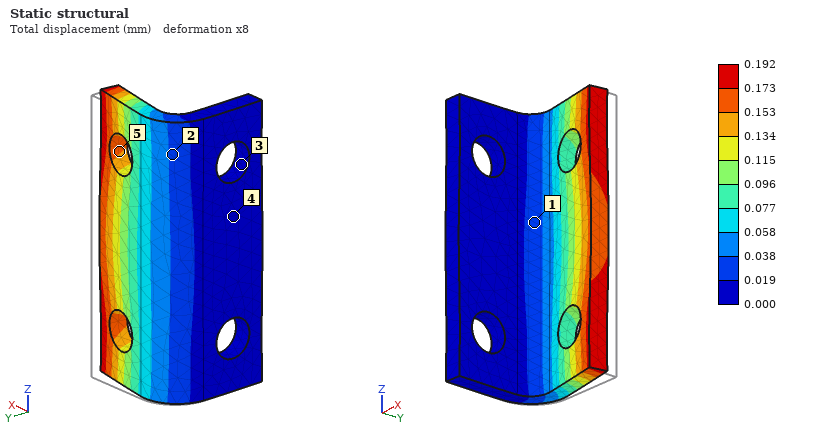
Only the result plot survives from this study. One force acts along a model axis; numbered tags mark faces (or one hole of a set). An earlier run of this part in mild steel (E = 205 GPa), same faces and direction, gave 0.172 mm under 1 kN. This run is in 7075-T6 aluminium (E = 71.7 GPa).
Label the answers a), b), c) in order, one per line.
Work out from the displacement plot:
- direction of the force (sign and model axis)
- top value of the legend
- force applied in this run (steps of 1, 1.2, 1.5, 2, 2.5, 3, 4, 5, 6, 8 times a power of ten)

a) -Y
b) 0.192 mm
c) 400 N
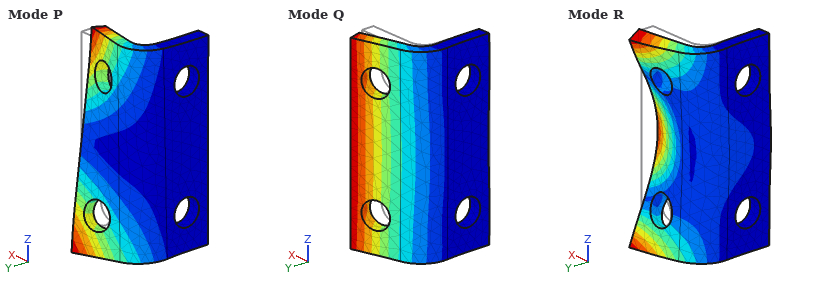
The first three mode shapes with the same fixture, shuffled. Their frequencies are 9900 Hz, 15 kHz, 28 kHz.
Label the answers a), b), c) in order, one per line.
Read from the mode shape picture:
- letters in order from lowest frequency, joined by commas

a) Q, P, R
